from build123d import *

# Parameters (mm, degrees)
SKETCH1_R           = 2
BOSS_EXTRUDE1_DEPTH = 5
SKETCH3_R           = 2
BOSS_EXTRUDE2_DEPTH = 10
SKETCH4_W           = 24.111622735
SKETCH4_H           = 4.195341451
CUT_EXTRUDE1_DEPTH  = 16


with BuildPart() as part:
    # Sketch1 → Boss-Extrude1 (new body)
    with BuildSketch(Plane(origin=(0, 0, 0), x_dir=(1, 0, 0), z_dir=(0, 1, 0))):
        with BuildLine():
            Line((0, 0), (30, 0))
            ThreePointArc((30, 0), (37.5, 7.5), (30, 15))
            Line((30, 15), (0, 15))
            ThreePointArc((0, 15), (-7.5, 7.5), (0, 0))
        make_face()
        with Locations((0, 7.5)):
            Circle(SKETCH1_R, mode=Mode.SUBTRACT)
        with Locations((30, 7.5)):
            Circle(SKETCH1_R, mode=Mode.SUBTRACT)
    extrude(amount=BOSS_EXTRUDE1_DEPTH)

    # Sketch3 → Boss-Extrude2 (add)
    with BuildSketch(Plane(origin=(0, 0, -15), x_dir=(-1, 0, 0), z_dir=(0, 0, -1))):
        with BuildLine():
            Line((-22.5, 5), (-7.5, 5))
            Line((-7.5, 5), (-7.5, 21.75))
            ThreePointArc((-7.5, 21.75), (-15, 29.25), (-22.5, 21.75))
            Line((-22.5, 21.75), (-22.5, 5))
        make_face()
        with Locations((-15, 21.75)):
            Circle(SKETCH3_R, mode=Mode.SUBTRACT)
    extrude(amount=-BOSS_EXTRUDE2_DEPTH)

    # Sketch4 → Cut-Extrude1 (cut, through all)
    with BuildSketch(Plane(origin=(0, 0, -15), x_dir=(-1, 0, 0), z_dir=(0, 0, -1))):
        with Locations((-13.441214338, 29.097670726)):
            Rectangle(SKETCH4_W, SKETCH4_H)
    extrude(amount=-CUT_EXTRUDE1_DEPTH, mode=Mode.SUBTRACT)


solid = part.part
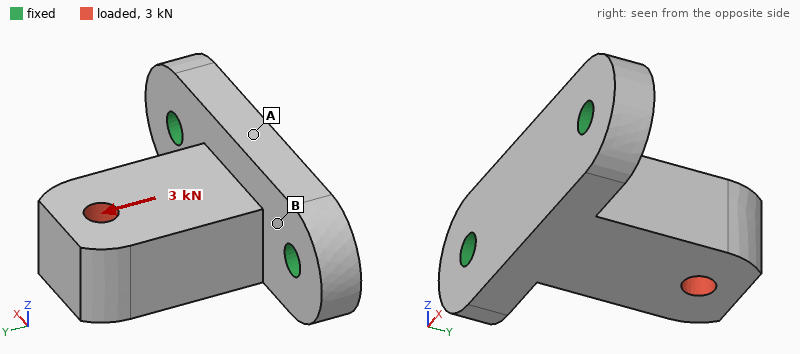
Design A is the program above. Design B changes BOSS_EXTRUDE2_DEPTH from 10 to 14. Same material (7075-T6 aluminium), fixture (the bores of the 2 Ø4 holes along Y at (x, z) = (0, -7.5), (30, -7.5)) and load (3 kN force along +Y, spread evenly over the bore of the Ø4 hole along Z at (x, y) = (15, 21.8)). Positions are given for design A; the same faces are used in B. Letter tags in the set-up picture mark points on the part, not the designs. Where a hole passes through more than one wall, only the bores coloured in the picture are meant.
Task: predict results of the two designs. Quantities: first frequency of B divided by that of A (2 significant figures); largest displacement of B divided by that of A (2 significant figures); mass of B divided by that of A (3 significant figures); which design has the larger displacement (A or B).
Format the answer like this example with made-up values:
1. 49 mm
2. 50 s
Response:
1. 0.94
2. 0.45
3. 1.20
4. A
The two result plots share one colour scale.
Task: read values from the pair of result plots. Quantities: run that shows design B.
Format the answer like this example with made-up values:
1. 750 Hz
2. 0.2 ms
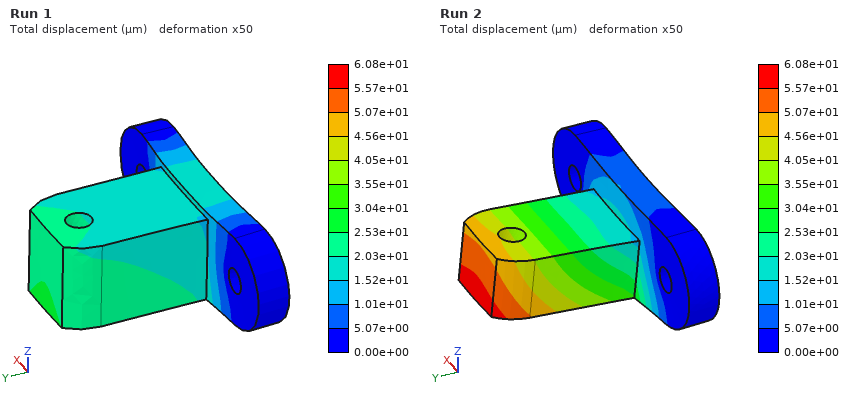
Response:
1. Run 1
